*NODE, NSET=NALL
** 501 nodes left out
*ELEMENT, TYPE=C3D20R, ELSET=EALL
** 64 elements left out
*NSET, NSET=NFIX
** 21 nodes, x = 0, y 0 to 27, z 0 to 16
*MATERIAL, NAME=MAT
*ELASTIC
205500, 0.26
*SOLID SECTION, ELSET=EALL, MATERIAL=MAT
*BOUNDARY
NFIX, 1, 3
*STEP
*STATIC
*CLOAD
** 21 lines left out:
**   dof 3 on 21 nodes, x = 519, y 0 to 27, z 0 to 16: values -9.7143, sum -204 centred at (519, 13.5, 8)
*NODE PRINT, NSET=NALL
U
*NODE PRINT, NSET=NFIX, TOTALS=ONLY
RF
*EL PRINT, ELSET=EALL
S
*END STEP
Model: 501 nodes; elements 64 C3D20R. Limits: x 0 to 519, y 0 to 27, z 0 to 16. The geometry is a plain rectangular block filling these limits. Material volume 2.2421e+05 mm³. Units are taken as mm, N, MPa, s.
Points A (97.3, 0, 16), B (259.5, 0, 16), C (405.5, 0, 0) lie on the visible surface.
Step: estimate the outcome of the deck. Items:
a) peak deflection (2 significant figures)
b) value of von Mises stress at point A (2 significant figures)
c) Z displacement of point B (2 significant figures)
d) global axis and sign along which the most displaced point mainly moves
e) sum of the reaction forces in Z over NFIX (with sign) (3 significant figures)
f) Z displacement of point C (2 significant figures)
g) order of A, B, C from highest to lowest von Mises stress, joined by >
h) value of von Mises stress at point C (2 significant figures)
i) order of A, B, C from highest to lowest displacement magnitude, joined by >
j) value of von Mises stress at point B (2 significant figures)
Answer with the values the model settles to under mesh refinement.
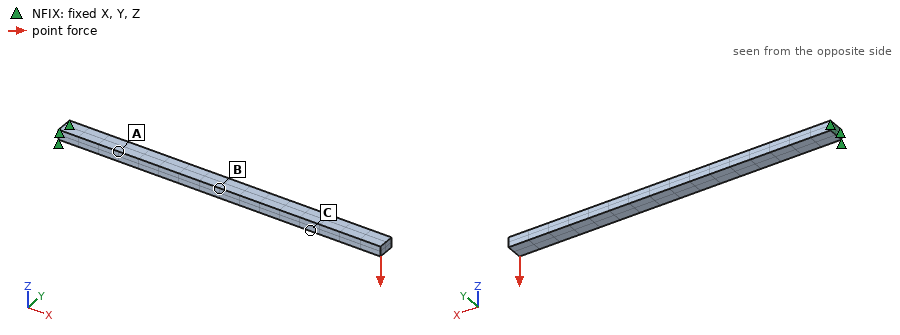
5.0 mm
75 MPa
-1.6 mm
-Z
204 N
-3.4 mm
A > B > C
20 MPa
C > B > A
46 MPa
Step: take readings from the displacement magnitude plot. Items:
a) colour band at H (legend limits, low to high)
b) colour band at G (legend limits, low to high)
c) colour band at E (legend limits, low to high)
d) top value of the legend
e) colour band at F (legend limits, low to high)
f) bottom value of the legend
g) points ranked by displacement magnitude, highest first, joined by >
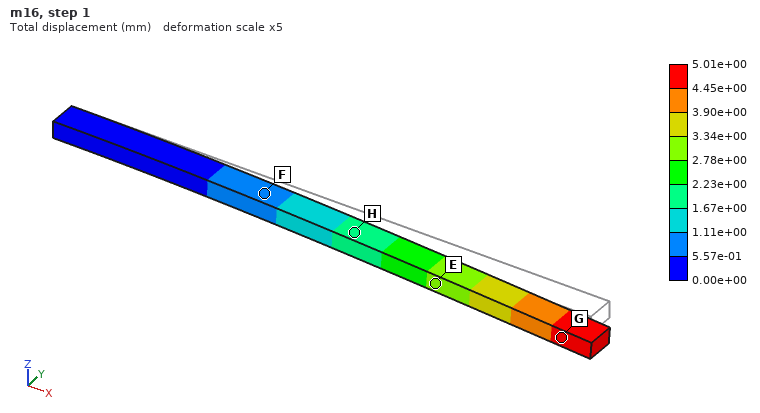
1.67e+00 to 2.23e+00 mm
4.45e+00 to 5.01e+00 mm
2.78e+00 to 3.34e+00 mm
5.01e+00 mm
5.57e-01 to 1.11e+00 mm
0.00e+00 mm
G > E > H > F
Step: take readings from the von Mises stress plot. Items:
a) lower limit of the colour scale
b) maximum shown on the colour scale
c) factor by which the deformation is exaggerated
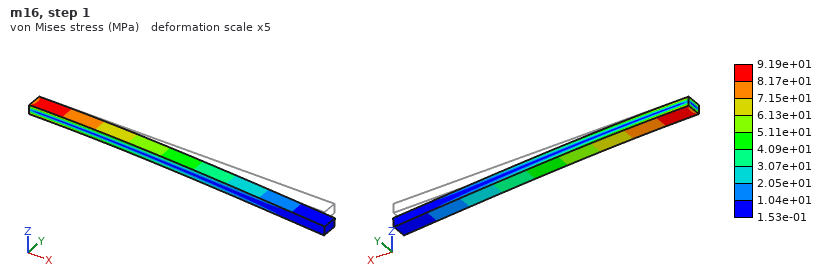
1.53e-01 MPa
9.19e+01 MPa
5
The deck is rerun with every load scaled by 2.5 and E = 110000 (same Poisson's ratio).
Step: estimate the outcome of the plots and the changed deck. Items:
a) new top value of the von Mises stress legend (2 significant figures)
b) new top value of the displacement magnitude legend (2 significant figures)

230 MPa
23 mm
